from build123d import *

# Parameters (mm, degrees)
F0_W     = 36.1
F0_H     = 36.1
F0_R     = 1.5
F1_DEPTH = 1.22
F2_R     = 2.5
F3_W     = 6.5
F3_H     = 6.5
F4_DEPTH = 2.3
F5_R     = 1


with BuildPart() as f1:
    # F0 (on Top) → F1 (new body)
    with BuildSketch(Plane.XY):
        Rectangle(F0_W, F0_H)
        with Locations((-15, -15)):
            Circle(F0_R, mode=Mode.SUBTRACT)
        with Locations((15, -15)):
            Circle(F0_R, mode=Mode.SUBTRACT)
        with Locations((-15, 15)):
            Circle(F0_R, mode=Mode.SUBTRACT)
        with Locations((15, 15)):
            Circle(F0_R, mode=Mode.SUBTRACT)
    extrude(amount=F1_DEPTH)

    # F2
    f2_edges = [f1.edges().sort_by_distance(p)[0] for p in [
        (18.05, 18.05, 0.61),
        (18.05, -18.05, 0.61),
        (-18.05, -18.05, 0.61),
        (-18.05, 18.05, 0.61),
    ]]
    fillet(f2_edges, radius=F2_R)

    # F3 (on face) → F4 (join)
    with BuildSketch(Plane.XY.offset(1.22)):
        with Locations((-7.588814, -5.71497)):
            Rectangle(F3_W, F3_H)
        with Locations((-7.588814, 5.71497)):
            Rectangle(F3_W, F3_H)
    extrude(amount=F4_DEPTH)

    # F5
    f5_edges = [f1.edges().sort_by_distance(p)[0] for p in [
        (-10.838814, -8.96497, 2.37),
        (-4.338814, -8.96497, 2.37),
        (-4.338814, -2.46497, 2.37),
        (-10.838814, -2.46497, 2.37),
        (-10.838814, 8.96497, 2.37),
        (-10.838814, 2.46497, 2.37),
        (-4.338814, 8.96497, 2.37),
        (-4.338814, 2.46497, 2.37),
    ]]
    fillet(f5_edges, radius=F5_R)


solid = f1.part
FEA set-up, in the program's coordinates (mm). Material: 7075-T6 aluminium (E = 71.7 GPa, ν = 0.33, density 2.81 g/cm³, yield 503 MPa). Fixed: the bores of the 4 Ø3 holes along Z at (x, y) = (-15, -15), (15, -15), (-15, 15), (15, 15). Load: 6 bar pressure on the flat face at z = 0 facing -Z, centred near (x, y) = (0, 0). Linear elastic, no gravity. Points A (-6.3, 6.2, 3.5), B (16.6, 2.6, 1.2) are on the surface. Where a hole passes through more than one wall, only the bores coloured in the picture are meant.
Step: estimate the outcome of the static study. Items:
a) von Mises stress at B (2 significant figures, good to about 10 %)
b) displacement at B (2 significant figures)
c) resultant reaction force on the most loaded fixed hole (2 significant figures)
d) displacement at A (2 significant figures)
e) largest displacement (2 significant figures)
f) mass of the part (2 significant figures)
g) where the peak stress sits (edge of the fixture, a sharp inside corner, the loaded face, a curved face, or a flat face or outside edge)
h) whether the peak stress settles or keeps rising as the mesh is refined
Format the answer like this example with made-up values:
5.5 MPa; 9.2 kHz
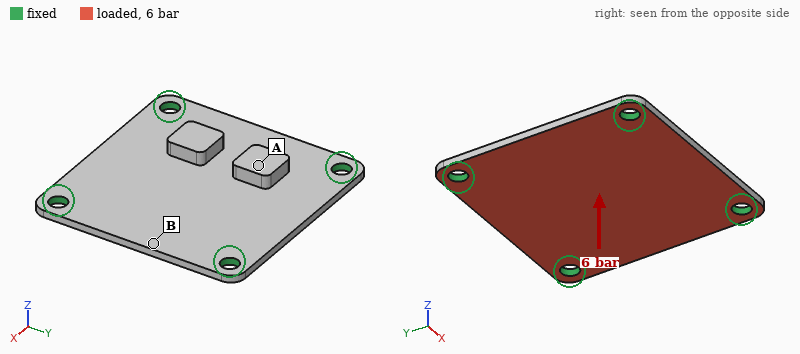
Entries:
93 MPa; 0.10 mm; 190 N; 0.17 mm; 0.24 mm; 4.9 g; edge of the fixture; keeps rising
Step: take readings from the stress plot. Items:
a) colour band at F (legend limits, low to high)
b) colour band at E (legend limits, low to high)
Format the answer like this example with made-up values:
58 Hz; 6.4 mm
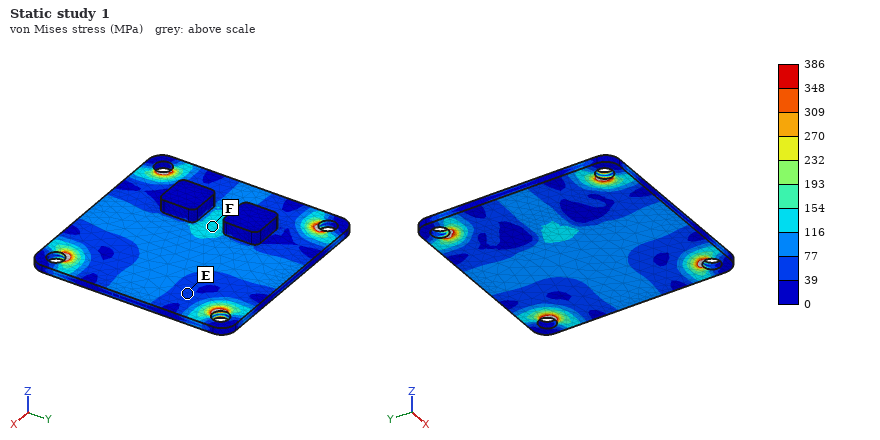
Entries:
116 to 154 MPa; 39 to 77 MPa
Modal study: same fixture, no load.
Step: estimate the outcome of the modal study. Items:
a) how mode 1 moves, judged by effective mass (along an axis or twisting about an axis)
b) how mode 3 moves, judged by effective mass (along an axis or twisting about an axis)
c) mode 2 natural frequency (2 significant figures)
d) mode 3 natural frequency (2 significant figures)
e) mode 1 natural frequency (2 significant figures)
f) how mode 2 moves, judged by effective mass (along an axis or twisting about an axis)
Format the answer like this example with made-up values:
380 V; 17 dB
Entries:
along Z; twisting about X; 8600 Hz; 9000 Hz; 4900 Hz; twisting about Y
